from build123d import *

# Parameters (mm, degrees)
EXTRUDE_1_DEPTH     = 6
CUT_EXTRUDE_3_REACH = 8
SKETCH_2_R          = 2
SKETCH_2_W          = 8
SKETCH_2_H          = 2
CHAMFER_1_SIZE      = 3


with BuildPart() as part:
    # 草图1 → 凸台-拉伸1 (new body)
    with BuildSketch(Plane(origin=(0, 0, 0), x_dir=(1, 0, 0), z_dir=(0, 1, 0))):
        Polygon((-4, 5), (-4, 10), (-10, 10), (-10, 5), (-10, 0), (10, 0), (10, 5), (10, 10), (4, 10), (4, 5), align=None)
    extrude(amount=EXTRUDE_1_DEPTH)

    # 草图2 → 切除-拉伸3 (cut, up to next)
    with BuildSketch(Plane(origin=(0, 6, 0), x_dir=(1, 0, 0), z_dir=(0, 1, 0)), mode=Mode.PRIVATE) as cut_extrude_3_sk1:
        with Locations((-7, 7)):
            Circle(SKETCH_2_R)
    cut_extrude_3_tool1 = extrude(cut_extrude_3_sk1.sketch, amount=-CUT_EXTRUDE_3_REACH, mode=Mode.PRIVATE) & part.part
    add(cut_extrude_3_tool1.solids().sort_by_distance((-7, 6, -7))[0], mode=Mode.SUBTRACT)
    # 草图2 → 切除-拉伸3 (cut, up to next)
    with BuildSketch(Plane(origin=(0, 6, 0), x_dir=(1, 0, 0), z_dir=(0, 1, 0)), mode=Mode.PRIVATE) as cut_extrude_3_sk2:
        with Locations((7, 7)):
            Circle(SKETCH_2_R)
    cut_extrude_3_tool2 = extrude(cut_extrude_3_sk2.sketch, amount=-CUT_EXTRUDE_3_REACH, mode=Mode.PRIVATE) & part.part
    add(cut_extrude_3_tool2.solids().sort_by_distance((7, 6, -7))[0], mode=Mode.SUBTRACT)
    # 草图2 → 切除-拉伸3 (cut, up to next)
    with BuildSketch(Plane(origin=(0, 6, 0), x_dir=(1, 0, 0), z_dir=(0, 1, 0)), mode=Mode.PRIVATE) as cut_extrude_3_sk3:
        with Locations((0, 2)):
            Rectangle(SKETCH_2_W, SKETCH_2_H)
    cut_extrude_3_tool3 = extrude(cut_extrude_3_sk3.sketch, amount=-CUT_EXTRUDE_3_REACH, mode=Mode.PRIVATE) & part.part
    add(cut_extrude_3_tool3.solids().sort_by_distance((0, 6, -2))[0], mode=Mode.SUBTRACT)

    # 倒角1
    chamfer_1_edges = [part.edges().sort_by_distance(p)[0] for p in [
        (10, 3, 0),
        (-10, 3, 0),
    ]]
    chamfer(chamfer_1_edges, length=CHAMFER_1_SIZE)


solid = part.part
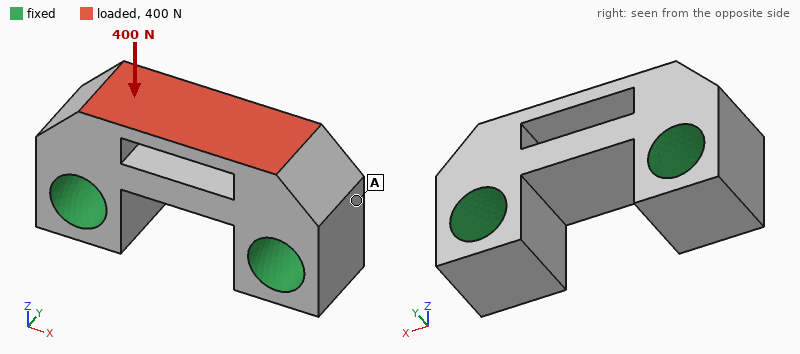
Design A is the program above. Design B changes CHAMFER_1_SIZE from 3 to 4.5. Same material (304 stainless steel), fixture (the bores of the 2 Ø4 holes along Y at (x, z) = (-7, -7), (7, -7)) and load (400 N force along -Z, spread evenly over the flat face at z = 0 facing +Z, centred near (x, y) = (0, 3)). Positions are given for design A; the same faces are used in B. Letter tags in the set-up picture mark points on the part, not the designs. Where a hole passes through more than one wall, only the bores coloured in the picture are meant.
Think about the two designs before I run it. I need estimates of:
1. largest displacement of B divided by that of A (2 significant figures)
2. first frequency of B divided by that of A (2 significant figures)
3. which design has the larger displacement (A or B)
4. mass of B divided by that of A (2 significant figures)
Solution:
1.3
0.99
B
0.90
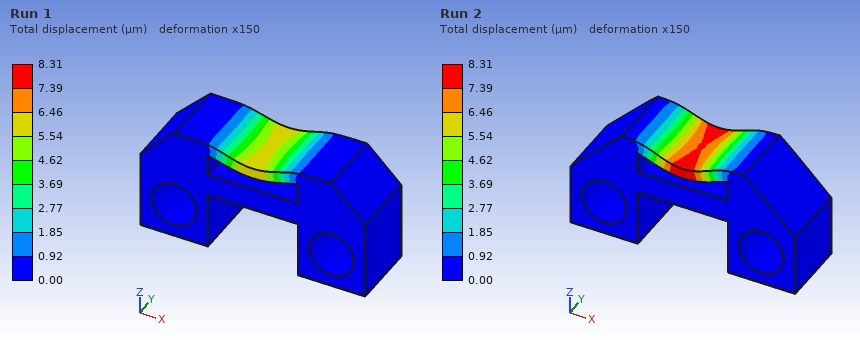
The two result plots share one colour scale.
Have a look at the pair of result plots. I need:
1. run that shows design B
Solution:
Run 2
